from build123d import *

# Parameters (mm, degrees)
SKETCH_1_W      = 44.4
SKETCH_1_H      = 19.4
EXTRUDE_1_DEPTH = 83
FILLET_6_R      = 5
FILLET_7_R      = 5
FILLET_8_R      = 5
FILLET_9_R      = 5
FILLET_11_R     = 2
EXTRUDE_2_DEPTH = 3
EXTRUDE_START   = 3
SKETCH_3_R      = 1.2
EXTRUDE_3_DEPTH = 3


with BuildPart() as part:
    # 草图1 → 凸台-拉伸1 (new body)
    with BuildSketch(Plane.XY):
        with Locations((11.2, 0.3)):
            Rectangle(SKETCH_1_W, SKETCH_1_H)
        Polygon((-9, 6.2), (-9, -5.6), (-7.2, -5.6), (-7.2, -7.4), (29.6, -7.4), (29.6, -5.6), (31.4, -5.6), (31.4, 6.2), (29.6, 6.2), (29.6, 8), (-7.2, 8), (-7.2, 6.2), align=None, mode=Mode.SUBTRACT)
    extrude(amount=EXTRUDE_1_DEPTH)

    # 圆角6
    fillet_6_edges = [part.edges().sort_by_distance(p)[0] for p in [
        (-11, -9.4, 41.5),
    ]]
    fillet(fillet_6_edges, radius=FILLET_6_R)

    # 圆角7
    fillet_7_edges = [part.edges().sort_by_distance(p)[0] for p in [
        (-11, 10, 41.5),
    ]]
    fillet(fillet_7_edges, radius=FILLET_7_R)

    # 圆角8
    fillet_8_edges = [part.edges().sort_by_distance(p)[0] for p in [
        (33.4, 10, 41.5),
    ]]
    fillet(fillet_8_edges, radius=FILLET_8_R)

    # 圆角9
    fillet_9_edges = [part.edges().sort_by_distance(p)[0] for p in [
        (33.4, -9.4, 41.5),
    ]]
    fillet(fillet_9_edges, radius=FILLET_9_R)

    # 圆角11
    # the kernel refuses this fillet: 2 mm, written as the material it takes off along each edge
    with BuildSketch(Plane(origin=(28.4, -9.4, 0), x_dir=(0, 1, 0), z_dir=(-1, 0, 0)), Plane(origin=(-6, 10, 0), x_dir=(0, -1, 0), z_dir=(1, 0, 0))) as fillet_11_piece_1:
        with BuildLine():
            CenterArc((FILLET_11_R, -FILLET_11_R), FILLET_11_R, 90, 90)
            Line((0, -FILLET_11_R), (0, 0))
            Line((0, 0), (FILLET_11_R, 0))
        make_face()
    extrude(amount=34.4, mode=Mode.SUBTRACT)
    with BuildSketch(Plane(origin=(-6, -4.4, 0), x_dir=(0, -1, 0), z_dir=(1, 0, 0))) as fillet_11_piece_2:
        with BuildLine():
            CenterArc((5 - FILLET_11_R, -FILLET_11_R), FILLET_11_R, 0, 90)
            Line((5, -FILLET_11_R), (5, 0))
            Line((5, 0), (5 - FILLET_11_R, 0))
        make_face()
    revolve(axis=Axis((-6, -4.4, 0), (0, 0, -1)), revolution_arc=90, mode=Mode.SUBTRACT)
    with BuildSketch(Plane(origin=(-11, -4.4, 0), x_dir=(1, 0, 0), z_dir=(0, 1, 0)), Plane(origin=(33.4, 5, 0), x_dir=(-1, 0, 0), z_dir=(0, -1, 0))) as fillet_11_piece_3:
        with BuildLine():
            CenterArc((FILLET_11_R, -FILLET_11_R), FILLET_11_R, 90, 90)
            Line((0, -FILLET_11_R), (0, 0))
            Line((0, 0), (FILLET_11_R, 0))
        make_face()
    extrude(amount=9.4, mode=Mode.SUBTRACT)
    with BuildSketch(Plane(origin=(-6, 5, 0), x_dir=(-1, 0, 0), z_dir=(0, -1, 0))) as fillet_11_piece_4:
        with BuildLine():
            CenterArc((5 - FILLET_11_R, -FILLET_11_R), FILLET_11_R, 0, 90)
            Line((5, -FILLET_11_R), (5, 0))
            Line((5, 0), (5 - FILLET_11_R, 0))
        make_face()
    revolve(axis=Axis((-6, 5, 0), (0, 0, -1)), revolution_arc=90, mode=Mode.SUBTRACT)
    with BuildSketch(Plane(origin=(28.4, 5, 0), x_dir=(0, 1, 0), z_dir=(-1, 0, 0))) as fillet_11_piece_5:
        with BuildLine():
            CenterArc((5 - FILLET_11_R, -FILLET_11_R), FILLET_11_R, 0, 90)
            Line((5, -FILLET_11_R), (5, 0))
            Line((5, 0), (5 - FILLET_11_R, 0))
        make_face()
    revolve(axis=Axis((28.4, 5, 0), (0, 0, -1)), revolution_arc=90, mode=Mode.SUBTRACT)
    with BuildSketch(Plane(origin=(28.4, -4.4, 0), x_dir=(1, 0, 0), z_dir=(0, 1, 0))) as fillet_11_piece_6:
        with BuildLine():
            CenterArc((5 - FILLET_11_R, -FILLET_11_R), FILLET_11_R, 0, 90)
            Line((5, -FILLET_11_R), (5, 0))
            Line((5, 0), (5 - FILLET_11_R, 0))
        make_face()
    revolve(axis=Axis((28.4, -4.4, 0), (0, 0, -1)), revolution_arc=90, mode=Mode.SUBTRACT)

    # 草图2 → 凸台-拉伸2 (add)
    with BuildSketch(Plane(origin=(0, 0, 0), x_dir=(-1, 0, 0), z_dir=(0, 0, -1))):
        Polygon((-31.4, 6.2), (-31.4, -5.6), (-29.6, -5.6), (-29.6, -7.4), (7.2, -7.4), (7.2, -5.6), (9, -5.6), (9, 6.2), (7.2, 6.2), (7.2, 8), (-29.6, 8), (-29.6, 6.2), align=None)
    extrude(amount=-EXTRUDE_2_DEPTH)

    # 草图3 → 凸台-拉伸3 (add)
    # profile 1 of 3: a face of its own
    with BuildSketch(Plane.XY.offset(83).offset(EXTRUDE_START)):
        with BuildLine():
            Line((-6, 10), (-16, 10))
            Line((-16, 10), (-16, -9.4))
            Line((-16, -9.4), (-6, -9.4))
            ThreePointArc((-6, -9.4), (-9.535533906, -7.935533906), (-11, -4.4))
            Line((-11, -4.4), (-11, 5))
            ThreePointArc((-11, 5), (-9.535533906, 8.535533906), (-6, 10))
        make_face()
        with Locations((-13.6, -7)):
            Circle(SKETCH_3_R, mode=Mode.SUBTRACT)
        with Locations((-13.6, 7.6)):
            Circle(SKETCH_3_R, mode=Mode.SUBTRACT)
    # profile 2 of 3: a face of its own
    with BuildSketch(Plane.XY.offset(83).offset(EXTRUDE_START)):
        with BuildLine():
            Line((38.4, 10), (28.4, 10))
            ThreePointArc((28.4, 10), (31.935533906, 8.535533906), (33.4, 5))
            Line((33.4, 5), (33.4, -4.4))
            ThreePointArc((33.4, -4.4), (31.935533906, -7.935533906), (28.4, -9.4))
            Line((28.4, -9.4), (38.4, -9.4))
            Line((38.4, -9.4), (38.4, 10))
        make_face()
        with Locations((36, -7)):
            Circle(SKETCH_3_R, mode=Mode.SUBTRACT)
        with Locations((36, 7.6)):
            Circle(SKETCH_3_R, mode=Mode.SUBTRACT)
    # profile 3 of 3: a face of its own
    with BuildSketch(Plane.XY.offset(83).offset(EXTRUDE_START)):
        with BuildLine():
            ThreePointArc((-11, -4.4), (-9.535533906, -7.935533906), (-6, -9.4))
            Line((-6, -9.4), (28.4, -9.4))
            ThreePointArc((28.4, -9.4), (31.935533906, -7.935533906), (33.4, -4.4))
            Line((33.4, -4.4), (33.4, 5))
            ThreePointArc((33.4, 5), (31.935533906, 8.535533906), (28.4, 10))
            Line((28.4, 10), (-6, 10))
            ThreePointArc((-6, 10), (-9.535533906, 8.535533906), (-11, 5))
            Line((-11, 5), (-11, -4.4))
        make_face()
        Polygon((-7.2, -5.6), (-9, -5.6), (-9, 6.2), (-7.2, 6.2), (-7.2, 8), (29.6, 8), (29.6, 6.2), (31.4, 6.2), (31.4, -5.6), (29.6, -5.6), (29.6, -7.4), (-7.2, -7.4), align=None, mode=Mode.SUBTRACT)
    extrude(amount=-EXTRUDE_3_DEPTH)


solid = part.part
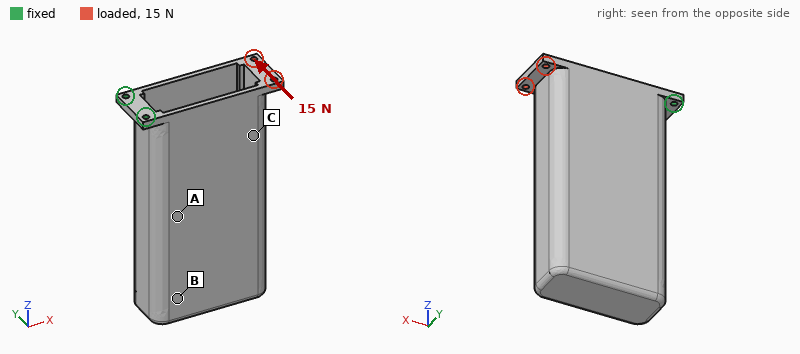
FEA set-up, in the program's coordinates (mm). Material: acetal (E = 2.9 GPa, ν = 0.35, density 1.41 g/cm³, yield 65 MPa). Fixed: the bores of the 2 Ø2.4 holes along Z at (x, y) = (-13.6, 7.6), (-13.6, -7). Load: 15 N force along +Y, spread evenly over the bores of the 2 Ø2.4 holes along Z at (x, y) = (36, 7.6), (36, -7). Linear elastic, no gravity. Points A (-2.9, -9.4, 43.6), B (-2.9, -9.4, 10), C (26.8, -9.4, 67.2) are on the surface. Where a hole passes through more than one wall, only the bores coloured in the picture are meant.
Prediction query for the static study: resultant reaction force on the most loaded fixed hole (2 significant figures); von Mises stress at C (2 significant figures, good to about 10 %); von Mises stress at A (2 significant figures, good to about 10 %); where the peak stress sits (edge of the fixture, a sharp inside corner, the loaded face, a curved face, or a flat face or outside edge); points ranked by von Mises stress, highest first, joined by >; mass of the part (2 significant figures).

46 N
3.6 MPa
2.0 MPa
a flat face or outside edge
C > A > B
31 g
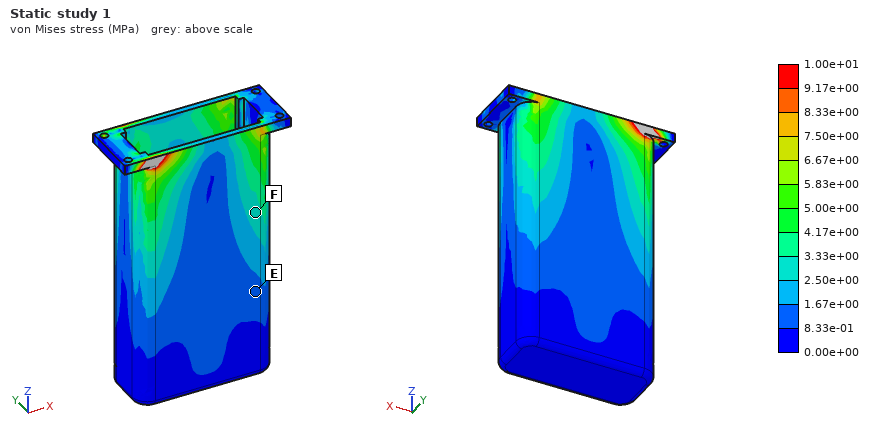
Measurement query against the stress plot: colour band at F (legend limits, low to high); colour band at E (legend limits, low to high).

2.50e+00 to 3.33e+00 MPa
8.33e-01 to 1.67e+00 MPa
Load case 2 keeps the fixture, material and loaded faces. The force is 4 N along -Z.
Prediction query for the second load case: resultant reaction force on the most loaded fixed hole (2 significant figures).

4.9 N
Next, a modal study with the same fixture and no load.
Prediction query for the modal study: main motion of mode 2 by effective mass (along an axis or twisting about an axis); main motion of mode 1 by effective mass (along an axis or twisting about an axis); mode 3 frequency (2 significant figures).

along Y
along X
300 Hz
